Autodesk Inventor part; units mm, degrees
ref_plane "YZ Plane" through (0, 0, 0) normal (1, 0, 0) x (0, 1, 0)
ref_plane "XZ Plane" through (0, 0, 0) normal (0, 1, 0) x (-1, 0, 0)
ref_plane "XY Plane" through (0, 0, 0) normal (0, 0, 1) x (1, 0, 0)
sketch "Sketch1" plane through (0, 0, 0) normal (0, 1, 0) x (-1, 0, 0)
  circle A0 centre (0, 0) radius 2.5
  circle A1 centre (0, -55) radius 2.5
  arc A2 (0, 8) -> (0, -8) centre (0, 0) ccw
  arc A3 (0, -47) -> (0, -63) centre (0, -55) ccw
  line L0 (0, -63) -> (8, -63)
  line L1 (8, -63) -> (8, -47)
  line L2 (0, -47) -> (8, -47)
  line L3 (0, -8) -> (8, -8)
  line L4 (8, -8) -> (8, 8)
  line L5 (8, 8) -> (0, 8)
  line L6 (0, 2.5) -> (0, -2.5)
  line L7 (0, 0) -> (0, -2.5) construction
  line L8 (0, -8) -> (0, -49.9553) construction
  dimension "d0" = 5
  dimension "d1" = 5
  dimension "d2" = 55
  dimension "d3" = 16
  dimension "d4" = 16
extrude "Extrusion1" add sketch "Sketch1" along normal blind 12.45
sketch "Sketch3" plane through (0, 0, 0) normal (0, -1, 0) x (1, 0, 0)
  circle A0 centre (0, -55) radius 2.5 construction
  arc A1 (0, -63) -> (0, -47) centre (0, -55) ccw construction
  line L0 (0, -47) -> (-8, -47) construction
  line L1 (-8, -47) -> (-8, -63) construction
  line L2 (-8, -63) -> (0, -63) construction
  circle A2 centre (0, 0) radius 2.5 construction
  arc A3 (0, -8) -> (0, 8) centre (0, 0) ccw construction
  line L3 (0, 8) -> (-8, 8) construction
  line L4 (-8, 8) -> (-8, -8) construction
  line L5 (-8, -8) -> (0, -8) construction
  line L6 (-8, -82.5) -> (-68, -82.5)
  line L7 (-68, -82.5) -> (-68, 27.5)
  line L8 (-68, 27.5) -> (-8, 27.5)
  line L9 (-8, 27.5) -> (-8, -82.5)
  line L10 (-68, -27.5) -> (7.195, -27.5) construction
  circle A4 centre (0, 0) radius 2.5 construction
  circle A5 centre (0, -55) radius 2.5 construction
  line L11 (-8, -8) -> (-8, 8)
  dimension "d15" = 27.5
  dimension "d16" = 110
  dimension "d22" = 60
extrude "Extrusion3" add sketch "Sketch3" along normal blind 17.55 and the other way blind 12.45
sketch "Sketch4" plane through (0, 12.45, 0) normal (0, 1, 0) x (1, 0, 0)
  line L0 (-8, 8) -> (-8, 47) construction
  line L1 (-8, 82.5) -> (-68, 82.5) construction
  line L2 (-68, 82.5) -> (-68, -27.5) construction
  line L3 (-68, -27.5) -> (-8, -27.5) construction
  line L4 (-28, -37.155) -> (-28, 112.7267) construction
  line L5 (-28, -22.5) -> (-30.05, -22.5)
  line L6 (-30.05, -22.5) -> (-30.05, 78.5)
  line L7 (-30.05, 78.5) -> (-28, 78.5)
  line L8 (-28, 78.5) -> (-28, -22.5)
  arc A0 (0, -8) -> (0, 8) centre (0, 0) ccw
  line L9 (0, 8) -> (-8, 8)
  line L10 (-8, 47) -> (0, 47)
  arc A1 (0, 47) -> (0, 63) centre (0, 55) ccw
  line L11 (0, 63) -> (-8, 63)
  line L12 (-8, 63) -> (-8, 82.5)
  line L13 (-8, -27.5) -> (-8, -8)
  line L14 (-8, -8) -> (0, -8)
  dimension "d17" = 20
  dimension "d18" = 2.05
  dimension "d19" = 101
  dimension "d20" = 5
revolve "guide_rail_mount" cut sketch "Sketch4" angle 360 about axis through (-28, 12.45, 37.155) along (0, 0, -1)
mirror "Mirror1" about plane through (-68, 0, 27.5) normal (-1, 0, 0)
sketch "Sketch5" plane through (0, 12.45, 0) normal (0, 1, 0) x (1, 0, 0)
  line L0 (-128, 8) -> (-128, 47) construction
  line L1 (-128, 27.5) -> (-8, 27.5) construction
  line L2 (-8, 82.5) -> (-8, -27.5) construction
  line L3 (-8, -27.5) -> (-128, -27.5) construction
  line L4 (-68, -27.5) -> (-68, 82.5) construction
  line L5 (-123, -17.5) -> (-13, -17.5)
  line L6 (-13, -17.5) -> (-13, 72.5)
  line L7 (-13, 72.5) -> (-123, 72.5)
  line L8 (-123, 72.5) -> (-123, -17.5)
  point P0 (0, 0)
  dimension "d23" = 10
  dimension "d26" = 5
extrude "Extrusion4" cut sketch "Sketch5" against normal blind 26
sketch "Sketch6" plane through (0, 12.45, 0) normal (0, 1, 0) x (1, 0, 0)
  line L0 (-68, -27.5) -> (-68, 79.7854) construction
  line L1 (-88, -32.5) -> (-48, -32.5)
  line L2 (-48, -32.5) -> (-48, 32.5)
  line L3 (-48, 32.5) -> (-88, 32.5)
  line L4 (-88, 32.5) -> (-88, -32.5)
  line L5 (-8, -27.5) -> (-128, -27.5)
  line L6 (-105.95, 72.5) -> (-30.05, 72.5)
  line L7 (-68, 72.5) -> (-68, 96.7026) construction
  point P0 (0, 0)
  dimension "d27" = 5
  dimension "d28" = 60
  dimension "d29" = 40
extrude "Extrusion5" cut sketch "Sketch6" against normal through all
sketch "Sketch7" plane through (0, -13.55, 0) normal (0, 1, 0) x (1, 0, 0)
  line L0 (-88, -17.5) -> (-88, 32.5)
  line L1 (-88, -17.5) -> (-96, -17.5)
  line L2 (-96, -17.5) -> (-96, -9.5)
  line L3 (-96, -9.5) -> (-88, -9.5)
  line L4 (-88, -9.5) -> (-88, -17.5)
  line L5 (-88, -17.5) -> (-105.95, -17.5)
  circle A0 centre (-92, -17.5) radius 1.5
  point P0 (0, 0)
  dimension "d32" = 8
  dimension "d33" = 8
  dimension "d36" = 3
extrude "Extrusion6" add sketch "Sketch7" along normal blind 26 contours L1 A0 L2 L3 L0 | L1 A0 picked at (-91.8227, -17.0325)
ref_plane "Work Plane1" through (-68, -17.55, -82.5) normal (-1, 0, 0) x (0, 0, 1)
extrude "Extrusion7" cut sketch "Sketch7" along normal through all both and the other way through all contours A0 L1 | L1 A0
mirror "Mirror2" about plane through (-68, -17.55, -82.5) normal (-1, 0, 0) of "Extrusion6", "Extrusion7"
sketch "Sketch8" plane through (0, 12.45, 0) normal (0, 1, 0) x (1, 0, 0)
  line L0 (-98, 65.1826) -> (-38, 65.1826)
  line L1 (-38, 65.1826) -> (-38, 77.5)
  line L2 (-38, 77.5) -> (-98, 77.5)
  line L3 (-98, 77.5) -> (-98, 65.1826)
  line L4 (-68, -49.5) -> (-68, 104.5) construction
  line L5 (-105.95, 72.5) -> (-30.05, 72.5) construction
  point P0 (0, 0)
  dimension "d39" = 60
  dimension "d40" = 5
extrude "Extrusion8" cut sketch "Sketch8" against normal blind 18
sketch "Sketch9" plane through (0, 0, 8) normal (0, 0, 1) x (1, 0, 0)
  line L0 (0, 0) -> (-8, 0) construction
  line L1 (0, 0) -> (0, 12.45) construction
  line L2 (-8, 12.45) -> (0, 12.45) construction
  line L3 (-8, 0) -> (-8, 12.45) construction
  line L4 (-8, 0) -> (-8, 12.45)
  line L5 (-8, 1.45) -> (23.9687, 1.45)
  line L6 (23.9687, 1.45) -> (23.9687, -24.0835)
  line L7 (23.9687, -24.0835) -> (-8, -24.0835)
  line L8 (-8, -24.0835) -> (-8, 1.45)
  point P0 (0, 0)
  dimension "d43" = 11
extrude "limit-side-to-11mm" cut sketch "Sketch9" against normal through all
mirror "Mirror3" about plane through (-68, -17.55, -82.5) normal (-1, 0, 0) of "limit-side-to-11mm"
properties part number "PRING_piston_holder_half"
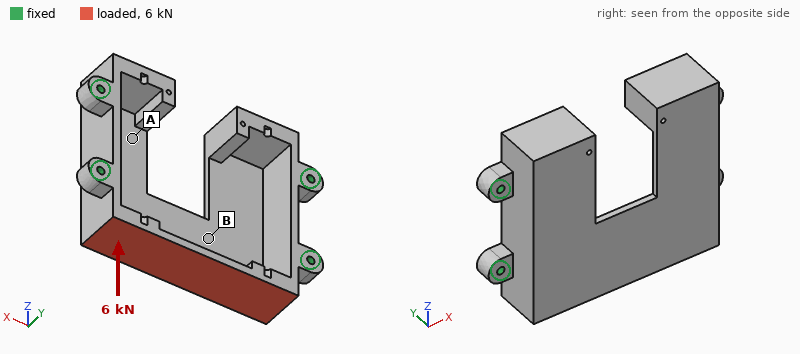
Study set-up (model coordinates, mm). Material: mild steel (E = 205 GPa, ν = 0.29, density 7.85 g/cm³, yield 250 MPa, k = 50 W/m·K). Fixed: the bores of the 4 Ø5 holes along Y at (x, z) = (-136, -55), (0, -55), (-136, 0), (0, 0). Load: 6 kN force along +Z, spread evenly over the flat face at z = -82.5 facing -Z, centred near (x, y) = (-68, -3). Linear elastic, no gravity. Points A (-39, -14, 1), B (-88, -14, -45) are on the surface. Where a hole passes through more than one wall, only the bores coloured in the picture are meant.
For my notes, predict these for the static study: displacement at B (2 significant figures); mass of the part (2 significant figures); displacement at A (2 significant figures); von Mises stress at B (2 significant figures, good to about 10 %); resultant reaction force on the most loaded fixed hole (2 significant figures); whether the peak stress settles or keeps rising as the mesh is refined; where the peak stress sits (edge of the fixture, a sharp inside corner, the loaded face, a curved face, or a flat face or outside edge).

19 µm
980 g
17 µm
16 MPa
2.3 kN
keeps rising
edge of the fixture
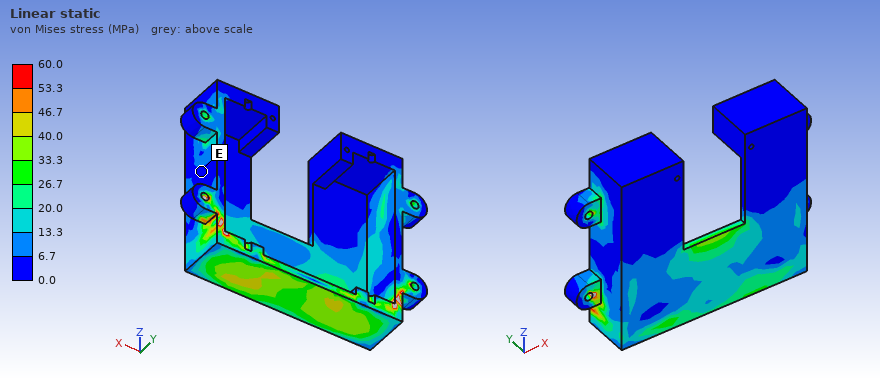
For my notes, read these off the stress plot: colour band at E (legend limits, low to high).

0.0 to 6.7 MPa
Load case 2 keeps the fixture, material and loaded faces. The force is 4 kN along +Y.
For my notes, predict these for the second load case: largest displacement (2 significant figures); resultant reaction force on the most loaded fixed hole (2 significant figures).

46 µm
3.1 kN
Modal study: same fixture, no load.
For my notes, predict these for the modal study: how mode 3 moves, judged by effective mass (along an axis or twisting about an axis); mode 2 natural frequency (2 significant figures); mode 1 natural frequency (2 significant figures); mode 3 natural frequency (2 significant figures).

along Y
2000 Hz
1900 Hz
3000 Hz
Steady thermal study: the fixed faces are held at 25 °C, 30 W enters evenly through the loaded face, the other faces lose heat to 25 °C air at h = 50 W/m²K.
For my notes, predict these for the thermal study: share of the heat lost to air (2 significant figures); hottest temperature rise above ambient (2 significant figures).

62 %
31 K
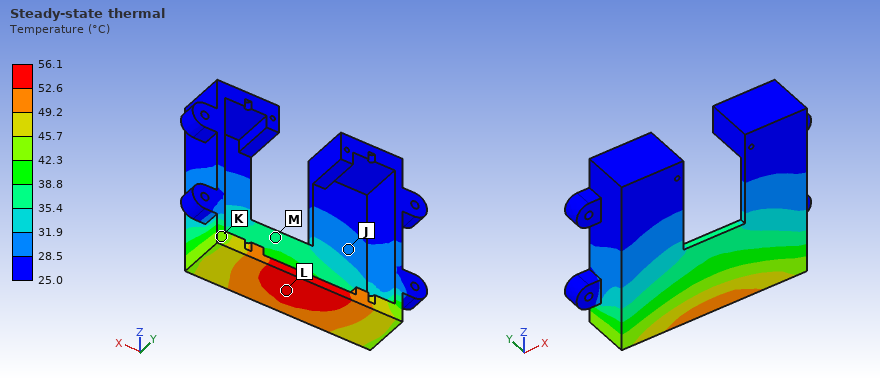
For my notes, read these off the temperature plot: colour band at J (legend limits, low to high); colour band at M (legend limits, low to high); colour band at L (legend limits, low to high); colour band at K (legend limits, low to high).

28.5 to 31.9 °C
35.4 to 38.8 °C
52.6 to 56.1 °C
42.3 to 45.7 °C
